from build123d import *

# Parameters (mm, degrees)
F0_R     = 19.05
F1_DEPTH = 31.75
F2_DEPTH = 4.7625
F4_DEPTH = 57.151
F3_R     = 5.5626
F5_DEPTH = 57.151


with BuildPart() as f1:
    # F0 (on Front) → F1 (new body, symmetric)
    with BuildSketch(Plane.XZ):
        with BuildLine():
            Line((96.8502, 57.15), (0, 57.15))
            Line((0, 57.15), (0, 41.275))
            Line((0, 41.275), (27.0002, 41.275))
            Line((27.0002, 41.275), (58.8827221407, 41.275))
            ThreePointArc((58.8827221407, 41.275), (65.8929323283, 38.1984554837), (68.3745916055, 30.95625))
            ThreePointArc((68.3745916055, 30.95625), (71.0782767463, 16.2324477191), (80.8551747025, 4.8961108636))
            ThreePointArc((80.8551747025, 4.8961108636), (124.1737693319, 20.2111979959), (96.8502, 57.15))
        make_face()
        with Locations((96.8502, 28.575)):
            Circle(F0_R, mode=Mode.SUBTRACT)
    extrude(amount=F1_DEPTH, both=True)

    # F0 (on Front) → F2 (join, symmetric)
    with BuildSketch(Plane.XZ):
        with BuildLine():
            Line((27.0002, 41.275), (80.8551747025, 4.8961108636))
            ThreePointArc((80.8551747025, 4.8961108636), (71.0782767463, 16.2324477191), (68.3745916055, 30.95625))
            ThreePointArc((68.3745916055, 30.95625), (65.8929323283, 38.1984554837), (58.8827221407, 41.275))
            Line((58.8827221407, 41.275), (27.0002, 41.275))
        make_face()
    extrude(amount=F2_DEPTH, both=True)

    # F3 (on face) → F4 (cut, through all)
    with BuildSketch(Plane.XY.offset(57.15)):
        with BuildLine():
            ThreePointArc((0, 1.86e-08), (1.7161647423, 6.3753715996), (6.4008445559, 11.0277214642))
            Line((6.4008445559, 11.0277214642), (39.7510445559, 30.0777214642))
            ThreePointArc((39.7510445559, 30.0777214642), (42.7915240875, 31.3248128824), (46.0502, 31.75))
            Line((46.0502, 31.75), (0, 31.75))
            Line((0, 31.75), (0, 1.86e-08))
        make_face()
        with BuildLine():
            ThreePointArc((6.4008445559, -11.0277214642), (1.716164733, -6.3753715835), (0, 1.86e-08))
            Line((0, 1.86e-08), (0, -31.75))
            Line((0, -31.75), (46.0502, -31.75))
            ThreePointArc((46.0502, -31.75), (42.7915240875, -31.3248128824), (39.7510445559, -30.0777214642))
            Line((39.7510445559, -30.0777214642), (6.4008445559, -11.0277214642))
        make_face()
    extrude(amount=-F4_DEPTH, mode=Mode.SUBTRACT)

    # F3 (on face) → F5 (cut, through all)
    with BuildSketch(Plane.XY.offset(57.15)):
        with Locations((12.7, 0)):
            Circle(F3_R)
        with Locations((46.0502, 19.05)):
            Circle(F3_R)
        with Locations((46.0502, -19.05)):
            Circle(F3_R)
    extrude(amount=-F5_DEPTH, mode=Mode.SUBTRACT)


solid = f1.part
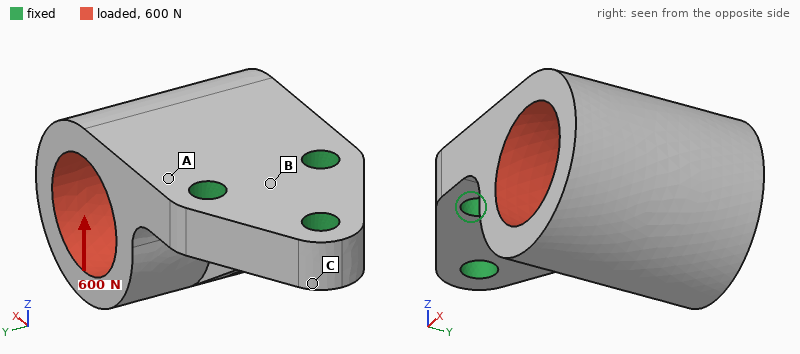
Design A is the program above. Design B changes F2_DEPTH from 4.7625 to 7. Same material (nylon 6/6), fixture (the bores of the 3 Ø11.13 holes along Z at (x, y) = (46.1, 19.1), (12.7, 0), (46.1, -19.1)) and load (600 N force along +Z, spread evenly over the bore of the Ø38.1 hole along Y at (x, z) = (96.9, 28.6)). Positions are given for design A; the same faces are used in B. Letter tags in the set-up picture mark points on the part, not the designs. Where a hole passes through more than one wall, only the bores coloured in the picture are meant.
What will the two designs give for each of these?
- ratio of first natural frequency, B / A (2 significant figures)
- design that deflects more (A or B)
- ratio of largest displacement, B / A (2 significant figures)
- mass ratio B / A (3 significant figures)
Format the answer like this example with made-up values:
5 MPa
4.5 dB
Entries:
1.0
A
0.91
1.02
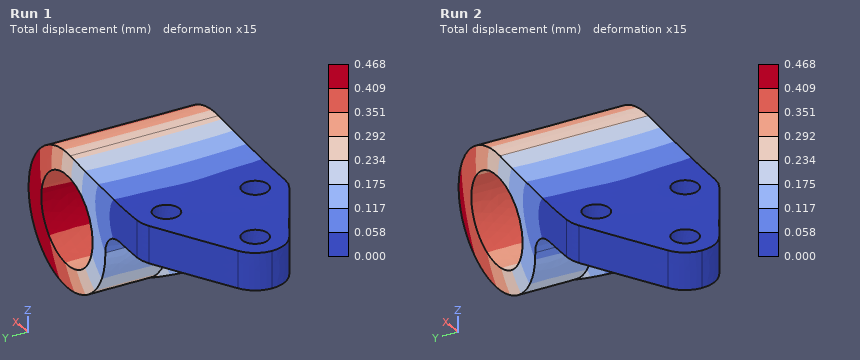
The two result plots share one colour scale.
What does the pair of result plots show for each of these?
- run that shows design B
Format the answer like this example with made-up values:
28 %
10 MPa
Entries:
Run 2
